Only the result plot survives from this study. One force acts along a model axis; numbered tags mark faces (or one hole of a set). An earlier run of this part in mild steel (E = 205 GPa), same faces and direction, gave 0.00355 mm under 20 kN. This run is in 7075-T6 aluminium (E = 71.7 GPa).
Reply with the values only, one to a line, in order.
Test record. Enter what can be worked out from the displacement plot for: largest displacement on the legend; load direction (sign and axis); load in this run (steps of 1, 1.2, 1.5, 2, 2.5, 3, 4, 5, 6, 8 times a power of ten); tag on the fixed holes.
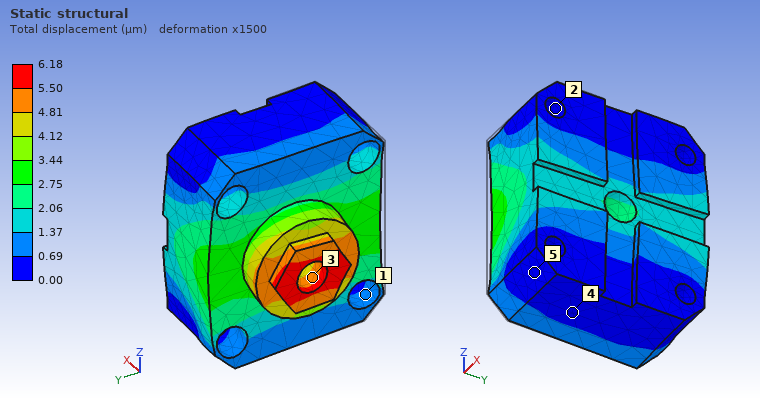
6.18 µm
+Y
12 kN
2
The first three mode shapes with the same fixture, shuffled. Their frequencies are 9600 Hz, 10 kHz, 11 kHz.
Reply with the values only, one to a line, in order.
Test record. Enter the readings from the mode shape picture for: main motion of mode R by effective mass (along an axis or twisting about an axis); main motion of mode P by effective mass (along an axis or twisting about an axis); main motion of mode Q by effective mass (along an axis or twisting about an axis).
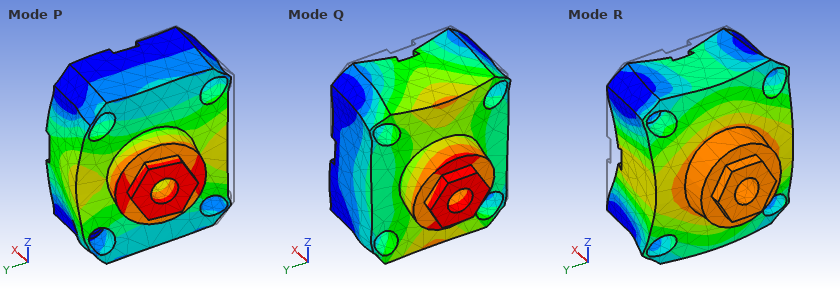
along X
along Y
along Z
